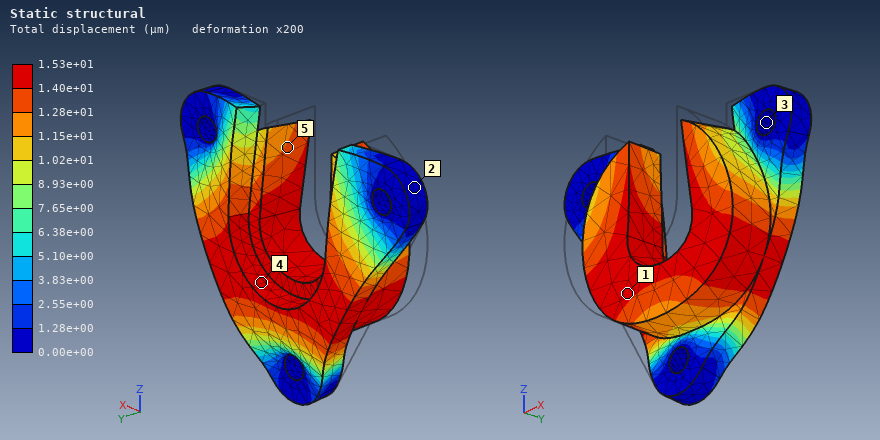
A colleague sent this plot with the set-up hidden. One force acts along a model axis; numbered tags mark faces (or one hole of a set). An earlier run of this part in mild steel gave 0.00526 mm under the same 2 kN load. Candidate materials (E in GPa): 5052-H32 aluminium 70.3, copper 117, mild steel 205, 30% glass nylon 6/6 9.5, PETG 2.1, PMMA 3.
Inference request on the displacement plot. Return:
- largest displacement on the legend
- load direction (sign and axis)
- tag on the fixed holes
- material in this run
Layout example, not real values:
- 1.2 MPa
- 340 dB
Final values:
- 1.53e+01 µm
- +Y
- 3
- 5052-H32 aluminium
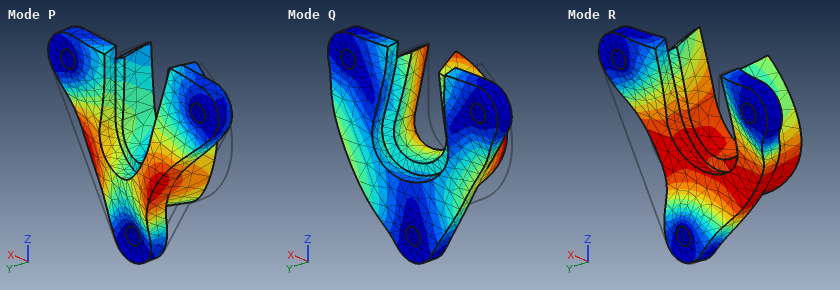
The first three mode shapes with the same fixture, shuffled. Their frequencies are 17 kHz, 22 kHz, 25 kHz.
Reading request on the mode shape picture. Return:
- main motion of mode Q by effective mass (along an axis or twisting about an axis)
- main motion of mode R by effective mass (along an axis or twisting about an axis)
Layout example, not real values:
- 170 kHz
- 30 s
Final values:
- along X
- along Y
